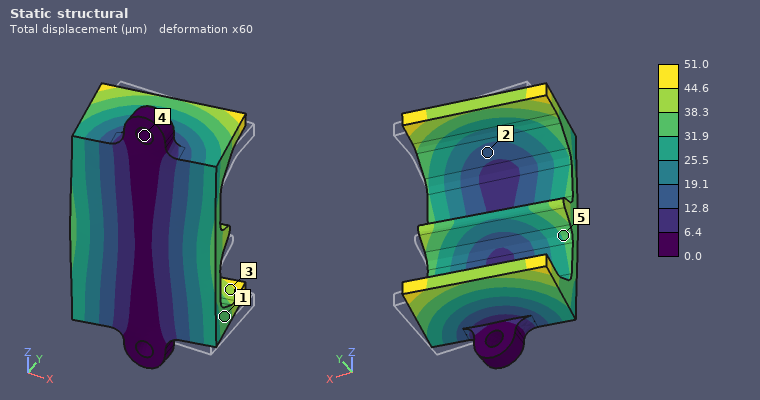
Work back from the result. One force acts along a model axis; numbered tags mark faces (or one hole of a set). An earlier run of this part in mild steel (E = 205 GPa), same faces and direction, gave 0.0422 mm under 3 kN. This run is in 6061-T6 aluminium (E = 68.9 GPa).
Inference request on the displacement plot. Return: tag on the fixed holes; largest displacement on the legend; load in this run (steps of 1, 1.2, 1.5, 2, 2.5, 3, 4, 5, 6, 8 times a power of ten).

4
51.0 µm
1.2 kN
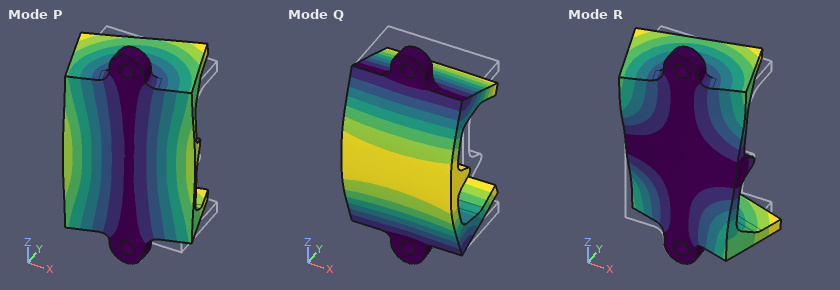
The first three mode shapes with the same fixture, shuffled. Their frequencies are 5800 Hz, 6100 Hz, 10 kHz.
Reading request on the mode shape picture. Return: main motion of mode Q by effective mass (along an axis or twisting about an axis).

along Y
